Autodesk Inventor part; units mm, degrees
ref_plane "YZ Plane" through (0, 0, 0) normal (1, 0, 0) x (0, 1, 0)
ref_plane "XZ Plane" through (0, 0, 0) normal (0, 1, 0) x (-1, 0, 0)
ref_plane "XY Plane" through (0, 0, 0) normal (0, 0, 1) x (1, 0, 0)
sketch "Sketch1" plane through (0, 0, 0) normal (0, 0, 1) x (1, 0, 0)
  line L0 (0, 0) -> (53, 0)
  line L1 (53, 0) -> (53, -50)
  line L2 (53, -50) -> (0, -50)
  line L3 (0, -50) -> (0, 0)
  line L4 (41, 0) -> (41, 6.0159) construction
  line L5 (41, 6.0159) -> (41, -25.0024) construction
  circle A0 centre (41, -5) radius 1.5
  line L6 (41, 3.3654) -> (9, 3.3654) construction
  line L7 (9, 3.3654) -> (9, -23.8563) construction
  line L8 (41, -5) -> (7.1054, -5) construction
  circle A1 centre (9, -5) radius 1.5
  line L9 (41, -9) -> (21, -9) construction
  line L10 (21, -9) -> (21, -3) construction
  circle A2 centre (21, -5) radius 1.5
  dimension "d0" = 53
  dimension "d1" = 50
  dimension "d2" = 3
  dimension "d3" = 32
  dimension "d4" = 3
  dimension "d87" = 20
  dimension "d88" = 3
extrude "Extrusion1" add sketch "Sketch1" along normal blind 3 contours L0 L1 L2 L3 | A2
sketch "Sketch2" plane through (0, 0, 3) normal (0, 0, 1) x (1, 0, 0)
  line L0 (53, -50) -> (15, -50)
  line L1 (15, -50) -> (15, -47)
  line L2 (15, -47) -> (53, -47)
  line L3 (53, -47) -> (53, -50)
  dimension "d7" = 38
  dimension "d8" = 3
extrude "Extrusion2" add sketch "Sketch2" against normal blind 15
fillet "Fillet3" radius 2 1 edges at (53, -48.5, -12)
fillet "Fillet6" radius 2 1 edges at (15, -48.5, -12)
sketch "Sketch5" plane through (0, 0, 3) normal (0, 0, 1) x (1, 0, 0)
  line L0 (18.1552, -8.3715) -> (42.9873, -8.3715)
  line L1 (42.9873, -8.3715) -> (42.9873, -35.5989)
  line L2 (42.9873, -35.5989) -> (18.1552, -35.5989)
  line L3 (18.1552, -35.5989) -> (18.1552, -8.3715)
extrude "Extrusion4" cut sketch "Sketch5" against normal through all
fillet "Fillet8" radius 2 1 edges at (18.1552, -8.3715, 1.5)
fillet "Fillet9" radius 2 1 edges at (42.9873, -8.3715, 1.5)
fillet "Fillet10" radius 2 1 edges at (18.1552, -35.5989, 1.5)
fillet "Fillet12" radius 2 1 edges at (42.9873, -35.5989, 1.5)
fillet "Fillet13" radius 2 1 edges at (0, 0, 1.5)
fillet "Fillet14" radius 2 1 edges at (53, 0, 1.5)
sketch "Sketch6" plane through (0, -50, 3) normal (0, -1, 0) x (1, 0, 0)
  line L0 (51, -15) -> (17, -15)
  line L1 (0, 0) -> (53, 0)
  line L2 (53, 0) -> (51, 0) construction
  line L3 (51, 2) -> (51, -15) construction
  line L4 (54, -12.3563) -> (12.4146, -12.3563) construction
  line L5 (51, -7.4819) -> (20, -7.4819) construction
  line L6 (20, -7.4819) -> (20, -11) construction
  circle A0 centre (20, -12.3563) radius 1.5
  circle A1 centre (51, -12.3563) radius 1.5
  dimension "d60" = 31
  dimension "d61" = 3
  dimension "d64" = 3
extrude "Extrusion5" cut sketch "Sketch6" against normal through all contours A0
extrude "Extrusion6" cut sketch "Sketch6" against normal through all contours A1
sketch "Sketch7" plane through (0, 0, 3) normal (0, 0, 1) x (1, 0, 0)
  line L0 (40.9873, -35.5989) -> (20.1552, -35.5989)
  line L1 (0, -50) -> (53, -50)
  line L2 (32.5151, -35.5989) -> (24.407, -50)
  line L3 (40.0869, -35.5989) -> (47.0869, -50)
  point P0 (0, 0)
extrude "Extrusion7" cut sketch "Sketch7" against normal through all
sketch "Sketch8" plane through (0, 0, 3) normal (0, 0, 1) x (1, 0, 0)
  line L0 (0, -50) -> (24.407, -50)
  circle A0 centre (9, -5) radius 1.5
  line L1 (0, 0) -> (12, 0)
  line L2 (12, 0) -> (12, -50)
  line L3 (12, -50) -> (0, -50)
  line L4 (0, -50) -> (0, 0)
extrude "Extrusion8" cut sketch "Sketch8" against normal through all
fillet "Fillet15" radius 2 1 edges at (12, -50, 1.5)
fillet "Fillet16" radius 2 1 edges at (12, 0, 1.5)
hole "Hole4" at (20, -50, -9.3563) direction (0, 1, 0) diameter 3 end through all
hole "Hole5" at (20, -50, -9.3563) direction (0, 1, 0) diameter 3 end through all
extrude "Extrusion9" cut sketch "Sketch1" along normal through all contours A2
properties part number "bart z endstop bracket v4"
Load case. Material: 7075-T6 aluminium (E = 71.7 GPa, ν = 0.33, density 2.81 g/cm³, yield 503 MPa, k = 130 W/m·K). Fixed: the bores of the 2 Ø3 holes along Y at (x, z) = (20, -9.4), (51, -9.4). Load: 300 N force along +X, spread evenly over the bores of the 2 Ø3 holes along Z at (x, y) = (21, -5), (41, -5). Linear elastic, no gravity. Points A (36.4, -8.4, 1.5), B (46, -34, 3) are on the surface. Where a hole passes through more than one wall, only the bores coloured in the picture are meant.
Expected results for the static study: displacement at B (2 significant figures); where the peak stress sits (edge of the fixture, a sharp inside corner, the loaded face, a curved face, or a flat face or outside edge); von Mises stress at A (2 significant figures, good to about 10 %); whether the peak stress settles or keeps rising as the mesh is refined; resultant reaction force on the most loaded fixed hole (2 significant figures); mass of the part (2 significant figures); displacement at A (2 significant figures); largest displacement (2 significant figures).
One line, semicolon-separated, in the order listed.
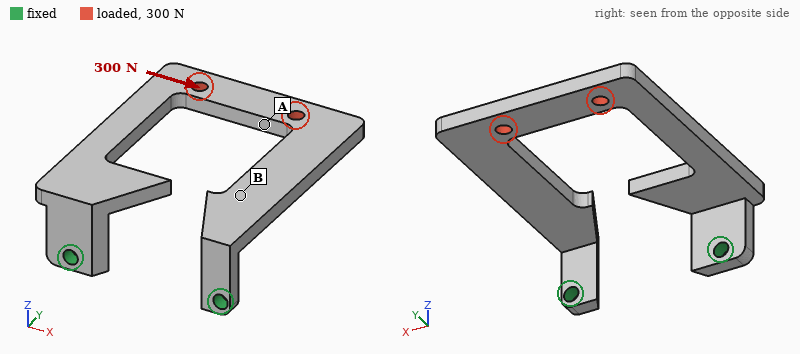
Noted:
0.22 mm; edge of the fixture; 72 MPa; keeps rising; 330 N; 11 g; 0.53 mm; 0.62 mm
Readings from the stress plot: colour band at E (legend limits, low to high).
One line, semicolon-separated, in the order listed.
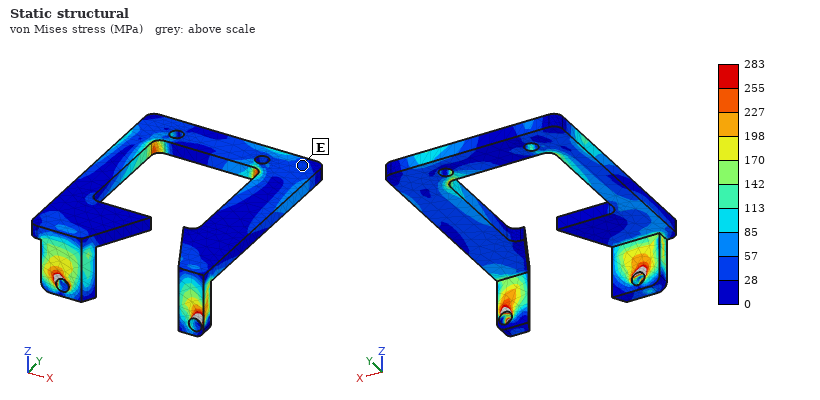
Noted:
28 to 57 MPa
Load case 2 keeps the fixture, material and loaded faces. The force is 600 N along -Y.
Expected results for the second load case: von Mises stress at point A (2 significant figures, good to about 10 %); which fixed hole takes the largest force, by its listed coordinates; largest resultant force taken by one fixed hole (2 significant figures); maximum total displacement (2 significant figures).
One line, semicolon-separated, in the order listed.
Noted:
44 MPa; (20, -9.4); 330 N; 0.61 mm
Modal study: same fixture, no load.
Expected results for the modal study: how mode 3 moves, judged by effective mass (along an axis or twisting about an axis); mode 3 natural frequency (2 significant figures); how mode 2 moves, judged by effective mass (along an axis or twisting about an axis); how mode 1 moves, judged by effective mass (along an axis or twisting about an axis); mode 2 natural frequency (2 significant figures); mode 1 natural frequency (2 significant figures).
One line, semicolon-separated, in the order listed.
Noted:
along X; 1900 Hz; along X; along Z; 1600 Hz; 610 Hz
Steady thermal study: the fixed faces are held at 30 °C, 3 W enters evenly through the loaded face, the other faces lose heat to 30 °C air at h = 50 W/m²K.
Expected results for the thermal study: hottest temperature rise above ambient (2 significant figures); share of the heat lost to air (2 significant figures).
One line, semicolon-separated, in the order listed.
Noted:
17 K; 48 %
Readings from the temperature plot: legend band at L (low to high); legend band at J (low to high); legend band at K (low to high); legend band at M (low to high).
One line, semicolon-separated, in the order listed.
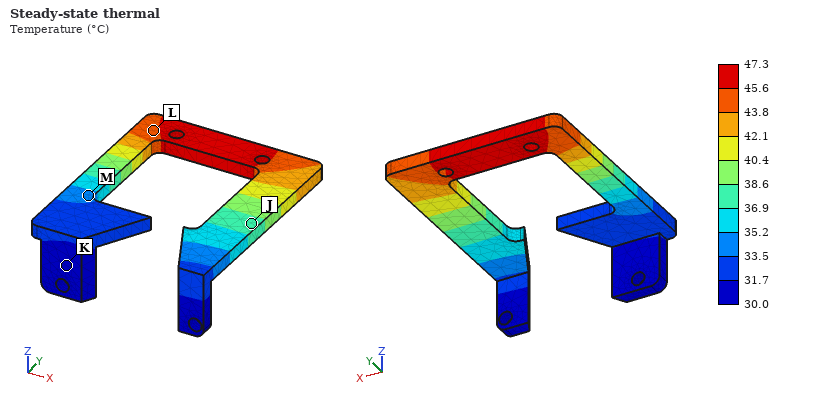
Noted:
43.8 to 45.6 °C; 36.9 to 38.6 °C; 30.0 to 31.7 °C; 33.5 to 35.2 °C
